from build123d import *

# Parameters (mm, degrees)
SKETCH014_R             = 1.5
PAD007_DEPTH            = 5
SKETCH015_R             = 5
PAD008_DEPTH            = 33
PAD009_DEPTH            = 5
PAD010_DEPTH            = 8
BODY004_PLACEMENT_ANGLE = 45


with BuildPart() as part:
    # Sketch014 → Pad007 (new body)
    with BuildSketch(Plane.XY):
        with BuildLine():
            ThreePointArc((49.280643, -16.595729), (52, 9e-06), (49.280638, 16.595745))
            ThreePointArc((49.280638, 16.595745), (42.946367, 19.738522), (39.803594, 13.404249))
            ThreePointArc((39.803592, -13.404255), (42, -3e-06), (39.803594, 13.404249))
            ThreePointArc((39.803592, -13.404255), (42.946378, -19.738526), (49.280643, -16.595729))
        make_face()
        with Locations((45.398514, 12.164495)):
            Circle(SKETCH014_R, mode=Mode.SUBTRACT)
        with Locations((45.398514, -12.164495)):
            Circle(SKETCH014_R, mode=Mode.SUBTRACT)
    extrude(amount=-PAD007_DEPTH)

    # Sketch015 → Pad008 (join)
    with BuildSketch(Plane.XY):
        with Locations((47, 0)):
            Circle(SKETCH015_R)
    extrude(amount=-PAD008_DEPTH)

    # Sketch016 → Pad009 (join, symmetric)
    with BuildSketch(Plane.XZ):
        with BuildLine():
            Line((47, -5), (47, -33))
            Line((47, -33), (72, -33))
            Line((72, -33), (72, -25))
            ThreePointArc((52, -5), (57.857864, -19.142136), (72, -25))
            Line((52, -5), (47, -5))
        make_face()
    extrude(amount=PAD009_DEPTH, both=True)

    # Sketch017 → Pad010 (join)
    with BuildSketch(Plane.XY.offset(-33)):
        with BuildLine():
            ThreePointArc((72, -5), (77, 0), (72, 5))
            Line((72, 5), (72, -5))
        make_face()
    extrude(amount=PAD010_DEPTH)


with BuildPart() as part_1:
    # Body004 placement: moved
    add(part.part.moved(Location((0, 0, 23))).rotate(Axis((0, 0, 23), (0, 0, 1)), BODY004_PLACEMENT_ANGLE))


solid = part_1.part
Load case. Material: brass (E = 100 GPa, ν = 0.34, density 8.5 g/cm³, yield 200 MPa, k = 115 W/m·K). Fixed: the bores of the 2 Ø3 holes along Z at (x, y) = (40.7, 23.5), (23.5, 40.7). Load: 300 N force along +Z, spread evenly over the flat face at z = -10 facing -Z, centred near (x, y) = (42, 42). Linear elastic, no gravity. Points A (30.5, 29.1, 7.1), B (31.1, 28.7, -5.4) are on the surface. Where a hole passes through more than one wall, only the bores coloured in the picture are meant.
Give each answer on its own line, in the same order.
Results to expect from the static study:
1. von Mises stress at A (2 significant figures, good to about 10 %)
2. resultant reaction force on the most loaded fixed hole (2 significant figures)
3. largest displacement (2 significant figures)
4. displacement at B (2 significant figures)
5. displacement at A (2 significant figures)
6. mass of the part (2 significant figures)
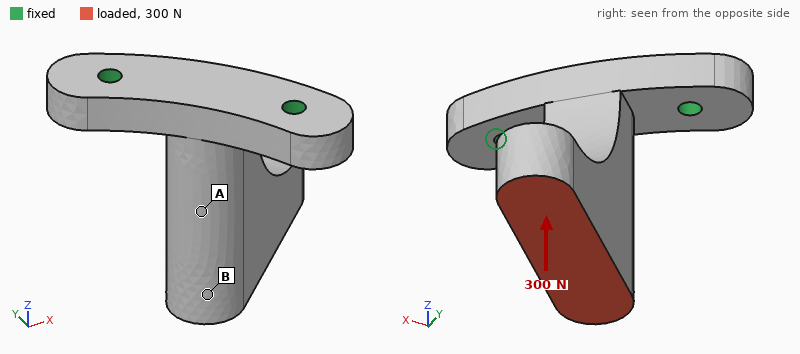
14 MPa
150 N
92 µm
50 µm
25 µm
61 g
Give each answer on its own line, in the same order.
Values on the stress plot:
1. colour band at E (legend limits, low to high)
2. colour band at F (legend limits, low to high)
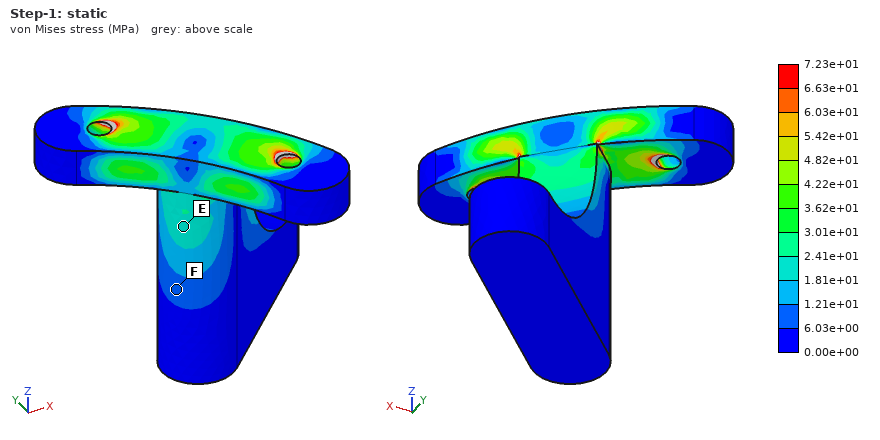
1.81e+01 to 2.41e+01 MPa
6.03e+00 to 1.21e+01 MPa
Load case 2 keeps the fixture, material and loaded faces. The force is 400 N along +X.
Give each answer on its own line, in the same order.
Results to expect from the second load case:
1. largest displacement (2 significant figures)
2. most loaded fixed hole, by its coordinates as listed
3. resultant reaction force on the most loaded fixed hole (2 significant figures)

0.21 mm
(23.5, 40.7)
620 N
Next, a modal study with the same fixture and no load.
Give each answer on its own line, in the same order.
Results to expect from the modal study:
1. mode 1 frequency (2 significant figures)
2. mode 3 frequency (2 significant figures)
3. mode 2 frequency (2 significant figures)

1400 Hz
5300 Hz
2300 Hz
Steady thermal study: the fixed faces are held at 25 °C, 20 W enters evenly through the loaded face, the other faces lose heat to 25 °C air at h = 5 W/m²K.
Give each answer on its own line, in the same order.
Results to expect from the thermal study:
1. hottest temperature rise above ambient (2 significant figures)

63 K
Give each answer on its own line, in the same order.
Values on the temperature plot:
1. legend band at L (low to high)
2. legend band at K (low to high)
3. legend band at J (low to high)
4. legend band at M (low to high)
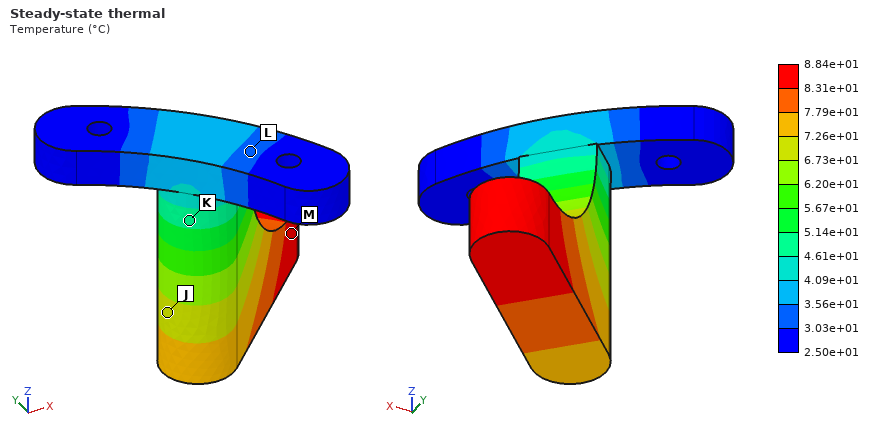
3.03e+01 to 3.56e+01 °C
4.61e+01 to 5.14e+01 °C
6.73e+01 to 7.26e+01 °C
8.31e+01 to 8.84e+01 °C
